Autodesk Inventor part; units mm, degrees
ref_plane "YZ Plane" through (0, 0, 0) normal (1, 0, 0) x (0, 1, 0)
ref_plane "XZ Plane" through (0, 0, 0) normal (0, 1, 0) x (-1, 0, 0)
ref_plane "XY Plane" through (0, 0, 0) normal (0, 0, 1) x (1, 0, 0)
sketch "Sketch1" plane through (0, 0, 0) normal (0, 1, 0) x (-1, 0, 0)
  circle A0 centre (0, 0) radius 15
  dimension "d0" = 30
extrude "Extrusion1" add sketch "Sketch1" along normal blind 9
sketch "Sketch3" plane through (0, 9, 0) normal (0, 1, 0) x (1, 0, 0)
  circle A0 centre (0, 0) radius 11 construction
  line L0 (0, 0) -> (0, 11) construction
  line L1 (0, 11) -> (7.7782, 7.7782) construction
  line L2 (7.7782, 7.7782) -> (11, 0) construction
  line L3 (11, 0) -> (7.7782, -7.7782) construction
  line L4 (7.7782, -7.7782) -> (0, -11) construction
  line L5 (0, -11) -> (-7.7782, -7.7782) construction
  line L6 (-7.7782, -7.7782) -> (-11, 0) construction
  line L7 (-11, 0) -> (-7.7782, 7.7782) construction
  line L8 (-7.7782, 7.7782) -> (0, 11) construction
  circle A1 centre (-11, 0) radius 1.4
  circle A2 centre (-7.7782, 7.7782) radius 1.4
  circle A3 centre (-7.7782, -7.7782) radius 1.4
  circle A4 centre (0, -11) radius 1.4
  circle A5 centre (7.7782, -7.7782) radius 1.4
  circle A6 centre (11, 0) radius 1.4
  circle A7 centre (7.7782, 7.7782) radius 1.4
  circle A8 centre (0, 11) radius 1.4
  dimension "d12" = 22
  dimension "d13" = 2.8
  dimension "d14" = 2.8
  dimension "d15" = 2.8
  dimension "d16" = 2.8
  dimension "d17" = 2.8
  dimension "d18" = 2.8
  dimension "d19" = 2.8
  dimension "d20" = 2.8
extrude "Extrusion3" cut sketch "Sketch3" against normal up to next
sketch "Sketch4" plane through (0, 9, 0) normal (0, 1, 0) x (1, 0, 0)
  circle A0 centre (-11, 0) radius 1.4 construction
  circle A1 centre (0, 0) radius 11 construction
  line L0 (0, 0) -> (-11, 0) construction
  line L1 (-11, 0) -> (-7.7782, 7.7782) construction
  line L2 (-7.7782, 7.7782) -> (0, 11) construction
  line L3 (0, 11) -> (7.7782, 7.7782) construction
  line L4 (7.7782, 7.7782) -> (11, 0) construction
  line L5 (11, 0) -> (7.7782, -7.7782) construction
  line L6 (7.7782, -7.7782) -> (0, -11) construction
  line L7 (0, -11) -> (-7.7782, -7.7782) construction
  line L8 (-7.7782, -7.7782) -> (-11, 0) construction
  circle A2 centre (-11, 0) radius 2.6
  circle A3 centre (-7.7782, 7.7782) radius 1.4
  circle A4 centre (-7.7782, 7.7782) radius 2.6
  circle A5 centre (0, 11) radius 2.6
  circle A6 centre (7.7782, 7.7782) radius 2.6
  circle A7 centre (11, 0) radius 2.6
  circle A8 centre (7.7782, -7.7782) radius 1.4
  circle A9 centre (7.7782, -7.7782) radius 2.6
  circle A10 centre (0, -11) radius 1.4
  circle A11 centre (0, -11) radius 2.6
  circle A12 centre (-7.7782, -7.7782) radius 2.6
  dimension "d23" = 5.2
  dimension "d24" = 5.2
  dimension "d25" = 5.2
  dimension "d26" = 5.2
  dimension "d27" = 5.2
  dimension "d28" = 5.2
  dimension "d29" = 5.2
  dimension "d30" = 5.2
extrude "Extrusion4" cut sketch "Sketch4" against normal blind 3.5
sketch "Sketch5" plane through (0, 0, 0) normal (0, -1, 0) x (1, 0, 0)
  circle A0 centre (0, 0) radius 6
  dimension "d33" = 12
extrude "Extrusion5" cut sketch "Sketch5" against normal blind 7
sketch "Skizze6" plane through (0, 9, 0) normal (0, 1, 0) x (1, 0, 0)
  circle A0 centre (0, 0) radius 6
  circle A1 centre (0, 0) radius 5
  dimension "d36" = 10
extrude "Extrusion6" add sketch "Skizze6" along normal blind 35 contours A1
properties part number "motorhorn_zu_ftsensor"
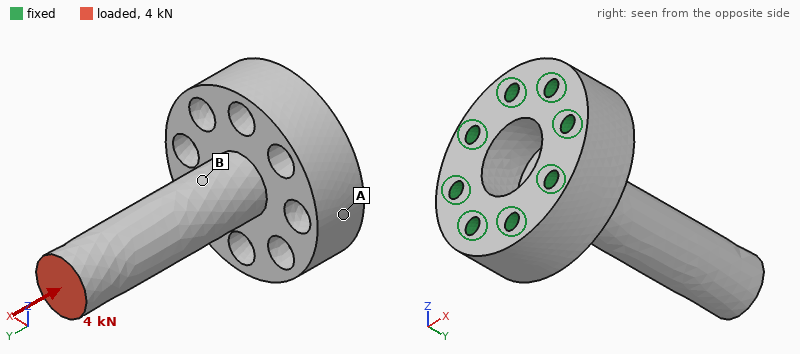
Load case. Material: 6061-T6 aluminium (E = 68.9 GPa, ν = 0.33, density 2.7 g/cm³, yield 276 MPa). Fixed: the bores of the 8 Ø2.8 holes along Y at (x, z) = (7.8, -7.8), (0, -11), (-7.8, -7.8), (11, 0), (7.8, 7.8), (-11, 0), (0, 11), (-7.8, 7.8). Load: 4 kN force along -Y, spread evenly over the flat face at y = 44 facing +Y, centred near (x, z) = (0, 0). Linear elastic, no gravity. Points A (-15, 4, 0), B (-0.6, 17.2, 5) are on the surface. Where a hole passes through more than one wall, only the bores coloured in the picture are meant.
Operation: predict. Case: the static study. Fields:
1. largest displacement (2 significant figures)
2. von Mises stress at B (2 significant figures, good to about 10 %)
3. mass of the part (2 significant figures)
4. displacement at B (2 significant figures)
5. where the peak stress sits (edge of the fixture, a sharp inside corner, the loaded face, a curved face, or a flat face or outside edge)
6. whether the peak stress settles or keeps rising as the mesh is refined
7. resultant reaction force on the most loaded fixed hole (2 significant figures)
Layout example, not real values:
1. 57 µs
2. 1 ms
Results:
1. 37 µm
2. 50 MPa
3. 20 g
4. 17 µm
5. a sharp inside corner
6. keeps rising
7. 670 N
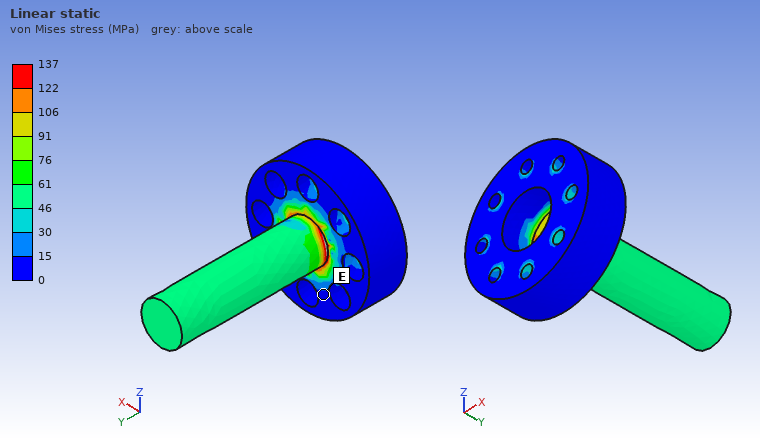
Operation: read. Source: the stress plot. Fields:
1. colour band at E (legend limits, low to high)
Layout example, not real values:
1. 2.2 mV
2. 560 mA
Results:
1. 0 to 15 MPa
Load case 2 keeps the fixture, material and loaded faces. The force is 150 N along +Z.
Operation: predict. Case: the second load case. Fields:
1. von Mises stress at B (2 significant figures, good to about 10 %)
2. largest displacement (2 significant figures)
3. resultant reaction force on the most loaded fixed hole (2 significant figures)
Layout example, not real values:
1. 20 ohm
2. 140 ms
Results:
1. 40 MPa
2. 98 µm
3. 190 N
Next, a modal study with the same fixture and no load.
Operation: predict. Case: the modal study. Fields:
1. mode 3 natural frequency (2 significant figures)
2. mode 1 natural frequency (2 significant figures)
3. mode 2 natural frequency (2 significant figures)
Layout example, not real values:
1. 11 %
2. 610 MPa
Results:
1. 21 kHz
2. 4400 Hz
3. 4400 Hz
